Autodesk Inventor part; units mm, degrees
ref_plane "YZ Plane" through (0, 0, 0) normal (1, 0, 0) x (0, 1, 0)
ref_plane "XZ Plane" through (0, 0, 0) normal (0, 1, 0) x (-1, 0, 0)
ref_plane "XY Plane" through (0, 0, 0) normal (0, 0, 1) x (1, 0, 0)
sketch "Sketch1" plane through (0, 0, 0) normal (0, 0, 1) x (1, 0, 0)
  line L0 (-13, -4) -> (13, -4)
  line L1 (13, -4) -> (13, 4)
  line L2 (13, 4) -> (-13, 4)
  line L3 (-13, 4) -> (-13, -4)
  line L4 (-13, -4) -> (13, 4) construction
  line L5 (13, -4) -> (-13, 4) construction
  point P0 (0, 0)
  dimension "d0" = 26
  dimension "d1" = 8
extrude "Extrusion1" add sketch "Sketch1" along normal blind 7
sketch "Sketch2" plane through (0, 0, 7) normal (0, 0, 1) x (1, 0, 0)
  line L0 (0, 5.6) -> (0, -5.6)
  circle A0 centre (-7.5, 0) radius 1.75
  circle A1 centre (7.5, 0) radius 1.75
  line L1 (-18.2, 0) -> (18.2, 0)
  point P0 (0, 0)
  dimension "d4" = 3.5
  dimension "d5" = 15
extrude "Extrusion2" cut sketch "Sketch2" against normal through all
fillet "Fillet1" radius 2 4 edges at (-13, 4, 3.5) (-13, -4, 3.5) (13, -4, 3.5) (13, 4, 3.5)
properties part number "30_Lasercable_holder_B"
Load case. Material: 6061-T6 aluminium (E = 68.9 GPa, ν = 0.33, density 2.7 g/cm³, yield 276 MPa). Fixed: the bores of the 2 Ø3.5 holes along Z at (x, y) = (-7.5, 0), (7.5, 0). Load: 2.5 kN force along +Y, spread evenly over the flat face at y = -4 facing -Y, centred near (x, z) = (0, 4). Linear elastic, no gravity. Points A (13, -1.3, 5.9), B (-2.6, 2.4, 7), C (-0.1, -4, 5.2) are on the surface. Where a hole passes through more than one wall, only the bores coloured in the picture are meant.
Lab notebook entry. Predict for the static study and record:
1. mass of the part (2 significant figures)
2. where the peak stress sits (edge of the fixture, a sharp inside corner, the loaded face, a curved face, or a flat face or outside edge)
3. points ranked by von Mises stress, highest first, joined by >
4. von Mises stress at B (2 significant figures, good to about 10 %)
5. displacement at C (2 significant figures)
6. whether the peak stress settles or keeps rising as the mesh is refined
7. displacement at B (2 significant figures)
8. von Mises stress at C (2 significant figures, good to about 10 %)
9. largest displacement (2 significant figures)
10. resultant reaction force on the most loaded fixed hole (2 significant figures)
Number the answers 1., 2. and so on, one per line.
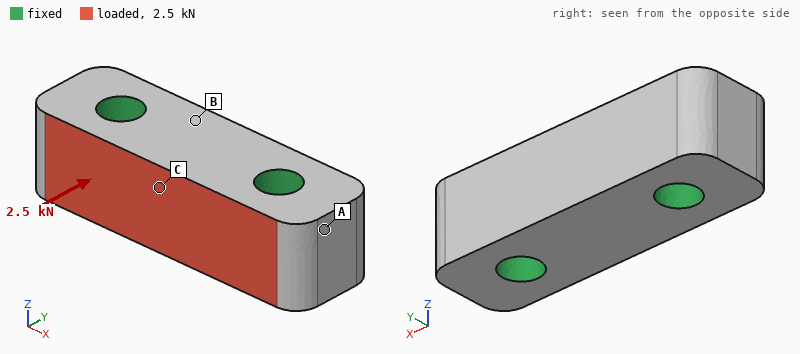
1. 3.5 g
2. edge of the fixture
3. C > B > A
4. 13 MPa
5. 3.1 µm
6. keeps rising
7. 2.0 µm
8. 22 MPa
9. 3.3 µm
10. 1.3 kN
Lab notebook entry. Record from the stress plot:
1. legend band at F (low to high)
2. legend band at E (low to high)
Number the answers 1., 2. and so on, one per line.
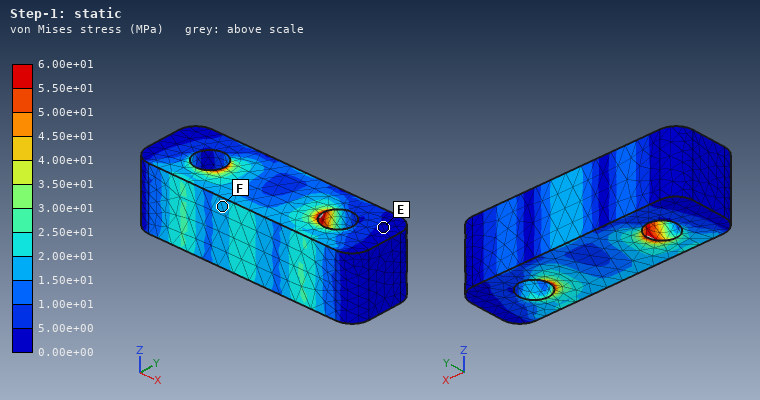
1. 1.50e+01 to 2.00e+01 MPa
2. 0.00e+00 to 5.00e+00 MPa
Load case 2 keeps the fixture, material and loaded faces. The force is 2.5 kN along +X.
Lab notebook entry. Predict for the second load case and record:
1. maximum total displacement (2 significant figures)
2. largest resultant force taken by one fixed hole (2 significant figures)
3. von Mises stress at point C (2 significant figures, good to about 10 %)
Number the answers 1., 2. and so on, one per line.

1. 2.6 µm
2. 1.3 kN
3. 28 MPa
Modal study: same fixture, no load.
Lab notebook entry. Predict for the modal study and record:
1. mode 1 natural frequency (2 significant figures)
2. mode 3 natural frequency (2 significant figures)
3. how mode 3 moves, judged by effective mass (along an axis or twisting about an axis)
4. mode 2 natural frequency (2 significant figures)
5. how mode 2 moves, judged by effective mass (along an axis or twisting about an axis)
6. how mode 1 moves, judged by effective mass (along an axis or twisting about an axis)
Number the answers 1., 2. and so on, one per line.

1. 91 kHz
2. 110 kHz
3. twisting about X
4. 97 kHz
5. along Z
6. along Y
